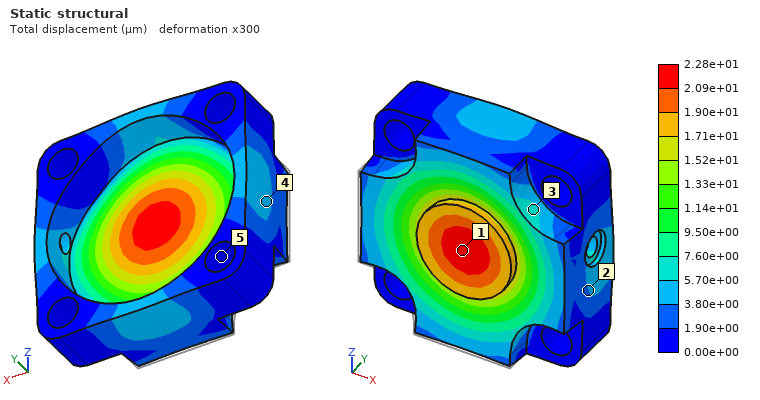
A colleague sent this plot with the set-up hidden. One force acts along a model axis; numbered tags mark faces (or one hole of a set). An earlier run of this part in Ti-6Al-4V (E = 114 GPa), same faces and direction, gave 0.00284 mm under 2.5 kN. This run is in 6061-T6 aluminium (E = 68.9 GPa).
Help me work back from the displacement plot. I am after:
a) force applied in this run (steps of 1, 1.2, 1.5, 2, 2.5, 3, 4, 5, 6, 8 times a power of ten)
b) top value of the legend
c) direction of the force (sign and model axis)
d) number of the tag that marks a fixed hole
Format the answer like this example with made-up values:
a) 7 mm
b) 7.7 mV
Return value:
a) 12 kN
b) 2.28e+01 µm
c) +Y
d) 5
